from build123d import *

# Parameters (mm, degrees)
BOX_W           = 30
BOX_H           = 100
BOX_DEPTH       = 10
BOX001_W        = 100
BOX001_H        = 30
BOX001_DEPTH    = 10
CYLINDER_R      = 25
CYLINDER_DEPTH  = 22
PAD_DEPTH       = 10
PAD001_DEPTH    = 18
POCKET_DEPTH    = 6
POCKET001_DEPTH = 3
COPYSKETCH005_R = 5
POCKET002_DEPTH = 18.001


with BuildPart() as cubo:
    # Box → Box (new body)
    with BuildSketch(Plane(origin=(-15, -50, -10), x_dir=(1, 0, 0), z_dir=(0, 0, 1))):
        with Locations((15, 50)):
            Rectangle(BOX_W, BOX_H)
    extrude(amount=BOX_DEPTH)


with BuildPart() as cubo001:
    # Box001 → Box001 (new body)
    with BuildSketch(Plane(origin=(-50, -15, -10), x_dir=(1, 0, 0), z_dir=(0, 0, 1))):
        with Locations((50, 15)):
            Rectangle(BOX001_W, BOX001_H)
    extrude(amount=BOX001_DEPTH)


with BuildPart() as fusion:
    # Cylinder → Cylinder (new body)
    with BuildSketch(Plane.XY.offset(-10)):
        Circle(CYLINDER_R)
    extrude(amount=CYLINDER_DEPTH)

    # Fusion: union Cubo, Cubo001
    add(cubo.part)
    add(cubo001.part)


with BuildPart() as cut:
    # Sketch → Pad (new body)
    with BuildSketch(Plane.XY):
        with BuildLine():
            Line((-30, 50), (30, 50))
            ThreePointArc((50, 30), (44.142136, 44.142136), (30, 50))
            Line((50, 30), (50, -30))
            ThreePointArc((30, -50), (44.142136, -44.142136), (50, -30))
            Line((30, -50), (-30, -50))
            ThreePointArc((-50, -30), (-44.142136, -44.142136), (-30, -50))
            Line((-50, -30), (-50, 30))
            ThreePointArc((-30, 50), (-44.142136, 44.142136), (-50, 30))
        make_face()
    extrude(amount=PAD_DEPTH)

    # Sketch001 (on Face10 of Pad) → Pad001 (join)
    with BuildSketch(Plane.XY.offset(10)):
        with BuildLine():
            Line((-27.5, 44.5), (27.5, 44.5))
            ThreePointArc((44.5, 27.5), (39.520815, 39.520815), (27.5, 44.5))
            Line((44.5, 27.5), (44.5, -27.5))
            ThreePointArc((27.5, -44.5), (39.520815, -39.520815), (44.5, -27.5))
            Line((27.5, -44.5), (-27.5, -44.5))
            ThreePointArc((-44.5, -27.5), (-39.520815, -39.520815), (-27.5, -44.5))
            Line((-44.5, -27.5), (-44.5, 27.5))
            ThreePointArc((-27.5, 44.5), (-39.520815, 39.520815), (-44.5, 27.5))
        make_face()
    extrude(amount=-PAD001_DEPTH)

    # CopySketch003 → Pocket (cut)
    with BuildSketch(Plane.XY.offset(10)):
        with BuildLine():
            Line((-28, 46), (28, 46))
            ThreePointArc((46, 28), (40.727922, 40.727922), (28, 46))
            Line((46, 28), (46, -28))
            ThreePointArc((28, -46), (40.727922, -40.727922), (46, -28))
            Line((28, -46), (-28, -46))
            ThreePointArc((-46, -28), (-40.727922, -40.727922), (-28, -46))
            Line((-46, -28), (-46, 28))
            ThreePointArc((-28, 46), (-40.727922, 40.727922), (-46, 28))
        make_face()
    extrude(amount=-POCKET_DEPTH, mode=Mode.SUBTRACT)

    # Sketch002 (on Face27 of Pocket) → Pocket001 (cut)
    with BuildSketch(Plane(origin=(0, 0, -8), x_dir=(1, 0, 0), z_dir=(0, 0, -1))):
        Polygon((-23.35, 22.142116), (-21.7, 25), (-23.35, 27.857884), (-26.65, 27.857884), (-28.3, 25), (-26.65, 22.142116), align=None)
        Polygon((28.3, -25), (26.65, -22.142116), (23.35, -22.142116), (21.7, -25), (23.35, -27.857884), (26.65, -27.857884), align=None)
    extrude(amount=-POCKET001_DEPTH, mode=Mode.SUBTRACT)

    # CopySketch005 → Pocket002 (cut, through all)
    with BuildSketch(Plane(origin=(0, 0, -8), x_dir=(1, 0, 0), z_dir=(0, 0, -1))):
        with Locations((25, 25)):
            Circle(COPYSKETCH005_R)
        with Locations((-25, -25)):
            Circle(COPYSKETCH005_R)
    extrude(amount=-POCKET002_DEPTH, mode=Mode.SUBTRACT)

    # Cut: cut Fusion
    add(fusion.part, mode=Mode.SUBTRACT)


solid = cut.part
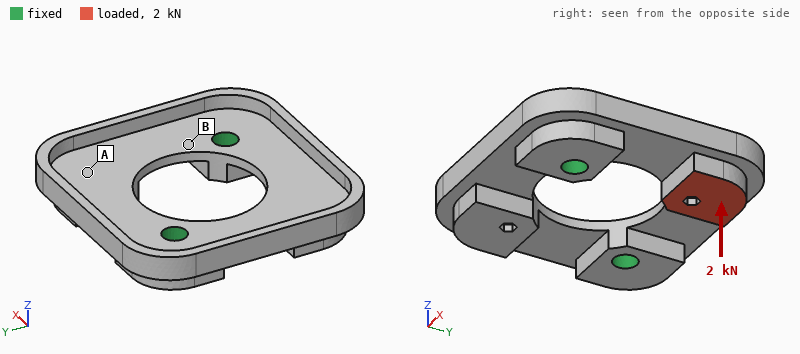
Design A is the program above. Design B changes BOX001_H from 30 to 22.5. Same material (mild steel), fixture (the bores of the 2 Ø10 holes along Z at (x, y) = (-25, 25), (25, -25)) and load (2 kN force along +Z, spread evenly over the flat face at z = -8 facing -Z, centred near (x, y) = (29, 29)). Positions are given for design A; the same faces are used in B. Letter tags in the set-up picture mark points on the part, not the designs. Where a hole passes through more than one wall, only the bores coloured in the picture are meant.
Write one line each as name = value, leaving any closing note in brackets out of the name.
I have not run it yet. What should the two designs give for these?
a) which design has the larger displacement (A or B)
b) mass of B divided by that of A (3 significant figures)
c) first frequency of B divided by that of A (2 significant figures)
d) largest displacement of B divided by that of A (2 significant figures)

which design has the larger displacement = A
mass of B divided by that of A = 1.04
first frequency of B divided by that of A = 1.1
largest displacement of B divided by that of A = 0.85
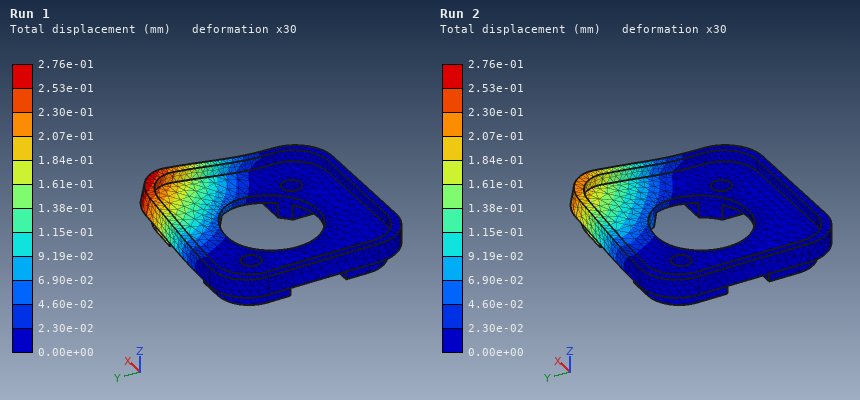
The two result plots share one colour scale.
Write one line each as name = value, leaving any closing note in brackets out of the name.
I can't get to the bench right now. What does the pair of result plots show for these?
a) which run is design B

which run is design B = Run 2
